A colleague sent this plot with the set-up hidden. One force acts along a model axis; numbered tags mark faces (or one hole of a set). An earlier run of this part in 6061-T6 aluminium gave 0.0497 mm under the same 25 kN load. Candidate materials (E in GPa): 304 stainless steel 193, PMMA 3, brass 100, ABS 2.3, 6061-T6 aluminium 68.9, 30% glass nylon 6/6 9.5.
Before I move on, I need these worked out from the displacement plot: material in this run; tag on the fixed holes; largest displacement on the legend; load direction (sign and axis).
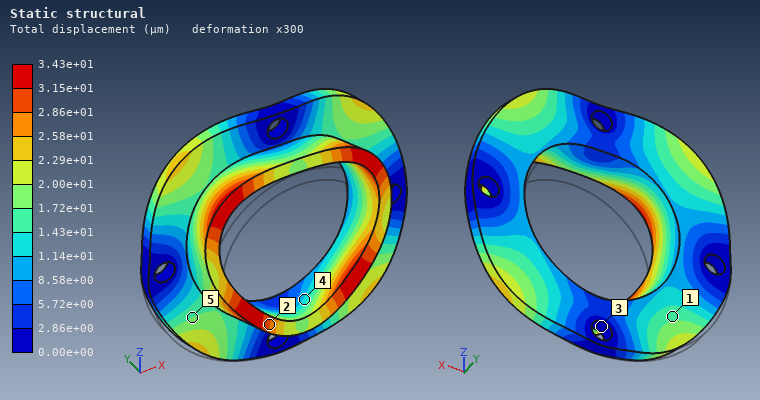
brass
3
3.43e+01 µm
+Z
